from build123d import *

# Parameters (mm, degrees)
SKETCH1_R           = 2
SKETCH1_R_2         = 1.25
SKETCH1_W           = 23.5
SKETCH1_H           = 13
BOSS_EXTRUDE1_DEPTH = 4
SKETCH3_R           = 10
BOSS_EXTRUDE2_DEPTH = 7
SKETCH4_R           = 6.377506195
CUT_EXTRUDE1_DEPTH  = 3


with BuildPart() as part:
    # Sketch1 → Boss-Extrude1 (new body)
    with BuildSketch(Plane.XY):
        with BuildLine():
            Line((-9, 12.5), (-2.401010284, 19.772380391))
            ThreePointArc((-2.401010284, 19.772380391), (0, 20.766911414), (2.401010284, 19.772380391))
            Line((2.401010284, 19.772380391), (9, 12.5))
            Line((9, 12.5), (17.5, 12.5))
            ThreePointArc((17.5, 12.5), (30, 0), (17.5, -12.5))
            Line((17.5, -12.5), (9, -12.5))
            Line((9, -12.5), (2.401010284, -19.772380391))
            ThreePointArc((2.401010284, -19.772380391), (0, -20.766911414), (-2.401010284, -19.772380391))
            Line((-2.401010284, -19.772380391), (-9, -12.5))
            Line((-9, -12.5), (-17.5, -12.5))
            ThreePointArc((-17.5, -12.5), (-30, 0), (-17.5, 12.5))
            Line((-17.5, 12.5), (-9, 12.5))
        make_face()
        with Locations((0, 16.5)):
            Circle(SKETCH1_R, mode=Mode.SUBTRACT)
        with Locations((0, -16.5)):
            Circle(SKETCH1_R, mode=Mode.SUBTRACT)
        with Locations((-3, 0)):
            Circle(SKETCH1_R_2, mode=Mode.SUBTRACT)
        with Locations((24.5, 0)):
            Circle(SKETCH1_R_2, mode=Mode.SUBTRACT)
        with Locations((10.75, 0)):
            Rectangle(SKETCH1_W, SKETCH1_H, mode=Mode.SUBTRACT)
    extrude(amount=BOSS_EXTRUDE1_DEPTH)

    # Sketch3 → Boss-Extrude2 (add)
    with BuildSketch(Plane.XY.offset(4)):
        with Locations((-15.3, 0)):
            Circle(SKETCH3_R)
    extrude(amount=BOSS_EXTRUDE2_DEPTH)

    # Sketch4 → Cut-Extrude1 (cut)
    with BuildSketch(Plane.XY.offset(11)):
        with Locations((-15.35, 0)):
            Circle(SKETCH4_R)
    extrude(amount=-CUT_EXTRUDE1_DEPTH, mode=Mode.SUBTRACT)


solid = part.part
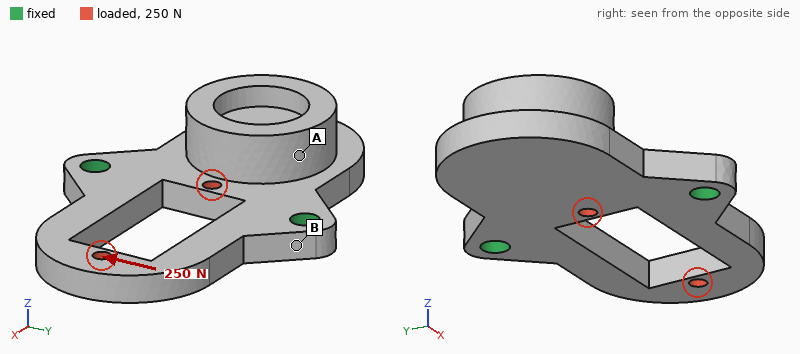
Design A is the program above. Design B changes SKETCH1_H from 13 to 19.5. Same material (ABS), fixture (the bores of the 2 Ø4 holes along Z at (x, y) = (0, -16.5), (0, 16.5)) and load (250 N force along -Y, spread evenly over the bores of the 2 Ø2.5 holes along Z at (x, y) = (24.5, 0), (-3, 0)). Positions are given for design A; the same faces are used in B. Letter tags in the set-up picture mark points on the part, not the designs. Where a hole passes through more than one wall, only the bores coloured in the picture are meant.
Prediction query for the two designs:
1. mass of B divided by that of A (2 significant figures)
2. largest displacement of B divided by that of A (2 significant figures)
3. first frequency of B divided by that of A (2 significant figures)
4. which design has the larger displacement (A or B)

0.91
5.9
0.95
B
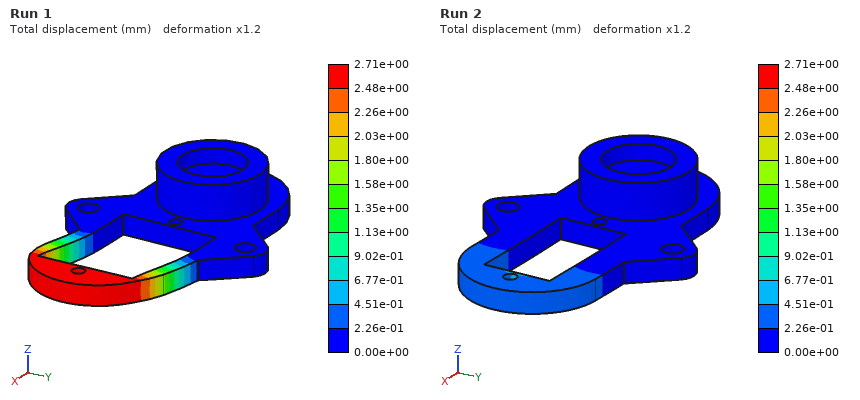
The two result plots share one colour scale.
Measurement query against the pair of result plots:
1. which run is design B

Run 1
